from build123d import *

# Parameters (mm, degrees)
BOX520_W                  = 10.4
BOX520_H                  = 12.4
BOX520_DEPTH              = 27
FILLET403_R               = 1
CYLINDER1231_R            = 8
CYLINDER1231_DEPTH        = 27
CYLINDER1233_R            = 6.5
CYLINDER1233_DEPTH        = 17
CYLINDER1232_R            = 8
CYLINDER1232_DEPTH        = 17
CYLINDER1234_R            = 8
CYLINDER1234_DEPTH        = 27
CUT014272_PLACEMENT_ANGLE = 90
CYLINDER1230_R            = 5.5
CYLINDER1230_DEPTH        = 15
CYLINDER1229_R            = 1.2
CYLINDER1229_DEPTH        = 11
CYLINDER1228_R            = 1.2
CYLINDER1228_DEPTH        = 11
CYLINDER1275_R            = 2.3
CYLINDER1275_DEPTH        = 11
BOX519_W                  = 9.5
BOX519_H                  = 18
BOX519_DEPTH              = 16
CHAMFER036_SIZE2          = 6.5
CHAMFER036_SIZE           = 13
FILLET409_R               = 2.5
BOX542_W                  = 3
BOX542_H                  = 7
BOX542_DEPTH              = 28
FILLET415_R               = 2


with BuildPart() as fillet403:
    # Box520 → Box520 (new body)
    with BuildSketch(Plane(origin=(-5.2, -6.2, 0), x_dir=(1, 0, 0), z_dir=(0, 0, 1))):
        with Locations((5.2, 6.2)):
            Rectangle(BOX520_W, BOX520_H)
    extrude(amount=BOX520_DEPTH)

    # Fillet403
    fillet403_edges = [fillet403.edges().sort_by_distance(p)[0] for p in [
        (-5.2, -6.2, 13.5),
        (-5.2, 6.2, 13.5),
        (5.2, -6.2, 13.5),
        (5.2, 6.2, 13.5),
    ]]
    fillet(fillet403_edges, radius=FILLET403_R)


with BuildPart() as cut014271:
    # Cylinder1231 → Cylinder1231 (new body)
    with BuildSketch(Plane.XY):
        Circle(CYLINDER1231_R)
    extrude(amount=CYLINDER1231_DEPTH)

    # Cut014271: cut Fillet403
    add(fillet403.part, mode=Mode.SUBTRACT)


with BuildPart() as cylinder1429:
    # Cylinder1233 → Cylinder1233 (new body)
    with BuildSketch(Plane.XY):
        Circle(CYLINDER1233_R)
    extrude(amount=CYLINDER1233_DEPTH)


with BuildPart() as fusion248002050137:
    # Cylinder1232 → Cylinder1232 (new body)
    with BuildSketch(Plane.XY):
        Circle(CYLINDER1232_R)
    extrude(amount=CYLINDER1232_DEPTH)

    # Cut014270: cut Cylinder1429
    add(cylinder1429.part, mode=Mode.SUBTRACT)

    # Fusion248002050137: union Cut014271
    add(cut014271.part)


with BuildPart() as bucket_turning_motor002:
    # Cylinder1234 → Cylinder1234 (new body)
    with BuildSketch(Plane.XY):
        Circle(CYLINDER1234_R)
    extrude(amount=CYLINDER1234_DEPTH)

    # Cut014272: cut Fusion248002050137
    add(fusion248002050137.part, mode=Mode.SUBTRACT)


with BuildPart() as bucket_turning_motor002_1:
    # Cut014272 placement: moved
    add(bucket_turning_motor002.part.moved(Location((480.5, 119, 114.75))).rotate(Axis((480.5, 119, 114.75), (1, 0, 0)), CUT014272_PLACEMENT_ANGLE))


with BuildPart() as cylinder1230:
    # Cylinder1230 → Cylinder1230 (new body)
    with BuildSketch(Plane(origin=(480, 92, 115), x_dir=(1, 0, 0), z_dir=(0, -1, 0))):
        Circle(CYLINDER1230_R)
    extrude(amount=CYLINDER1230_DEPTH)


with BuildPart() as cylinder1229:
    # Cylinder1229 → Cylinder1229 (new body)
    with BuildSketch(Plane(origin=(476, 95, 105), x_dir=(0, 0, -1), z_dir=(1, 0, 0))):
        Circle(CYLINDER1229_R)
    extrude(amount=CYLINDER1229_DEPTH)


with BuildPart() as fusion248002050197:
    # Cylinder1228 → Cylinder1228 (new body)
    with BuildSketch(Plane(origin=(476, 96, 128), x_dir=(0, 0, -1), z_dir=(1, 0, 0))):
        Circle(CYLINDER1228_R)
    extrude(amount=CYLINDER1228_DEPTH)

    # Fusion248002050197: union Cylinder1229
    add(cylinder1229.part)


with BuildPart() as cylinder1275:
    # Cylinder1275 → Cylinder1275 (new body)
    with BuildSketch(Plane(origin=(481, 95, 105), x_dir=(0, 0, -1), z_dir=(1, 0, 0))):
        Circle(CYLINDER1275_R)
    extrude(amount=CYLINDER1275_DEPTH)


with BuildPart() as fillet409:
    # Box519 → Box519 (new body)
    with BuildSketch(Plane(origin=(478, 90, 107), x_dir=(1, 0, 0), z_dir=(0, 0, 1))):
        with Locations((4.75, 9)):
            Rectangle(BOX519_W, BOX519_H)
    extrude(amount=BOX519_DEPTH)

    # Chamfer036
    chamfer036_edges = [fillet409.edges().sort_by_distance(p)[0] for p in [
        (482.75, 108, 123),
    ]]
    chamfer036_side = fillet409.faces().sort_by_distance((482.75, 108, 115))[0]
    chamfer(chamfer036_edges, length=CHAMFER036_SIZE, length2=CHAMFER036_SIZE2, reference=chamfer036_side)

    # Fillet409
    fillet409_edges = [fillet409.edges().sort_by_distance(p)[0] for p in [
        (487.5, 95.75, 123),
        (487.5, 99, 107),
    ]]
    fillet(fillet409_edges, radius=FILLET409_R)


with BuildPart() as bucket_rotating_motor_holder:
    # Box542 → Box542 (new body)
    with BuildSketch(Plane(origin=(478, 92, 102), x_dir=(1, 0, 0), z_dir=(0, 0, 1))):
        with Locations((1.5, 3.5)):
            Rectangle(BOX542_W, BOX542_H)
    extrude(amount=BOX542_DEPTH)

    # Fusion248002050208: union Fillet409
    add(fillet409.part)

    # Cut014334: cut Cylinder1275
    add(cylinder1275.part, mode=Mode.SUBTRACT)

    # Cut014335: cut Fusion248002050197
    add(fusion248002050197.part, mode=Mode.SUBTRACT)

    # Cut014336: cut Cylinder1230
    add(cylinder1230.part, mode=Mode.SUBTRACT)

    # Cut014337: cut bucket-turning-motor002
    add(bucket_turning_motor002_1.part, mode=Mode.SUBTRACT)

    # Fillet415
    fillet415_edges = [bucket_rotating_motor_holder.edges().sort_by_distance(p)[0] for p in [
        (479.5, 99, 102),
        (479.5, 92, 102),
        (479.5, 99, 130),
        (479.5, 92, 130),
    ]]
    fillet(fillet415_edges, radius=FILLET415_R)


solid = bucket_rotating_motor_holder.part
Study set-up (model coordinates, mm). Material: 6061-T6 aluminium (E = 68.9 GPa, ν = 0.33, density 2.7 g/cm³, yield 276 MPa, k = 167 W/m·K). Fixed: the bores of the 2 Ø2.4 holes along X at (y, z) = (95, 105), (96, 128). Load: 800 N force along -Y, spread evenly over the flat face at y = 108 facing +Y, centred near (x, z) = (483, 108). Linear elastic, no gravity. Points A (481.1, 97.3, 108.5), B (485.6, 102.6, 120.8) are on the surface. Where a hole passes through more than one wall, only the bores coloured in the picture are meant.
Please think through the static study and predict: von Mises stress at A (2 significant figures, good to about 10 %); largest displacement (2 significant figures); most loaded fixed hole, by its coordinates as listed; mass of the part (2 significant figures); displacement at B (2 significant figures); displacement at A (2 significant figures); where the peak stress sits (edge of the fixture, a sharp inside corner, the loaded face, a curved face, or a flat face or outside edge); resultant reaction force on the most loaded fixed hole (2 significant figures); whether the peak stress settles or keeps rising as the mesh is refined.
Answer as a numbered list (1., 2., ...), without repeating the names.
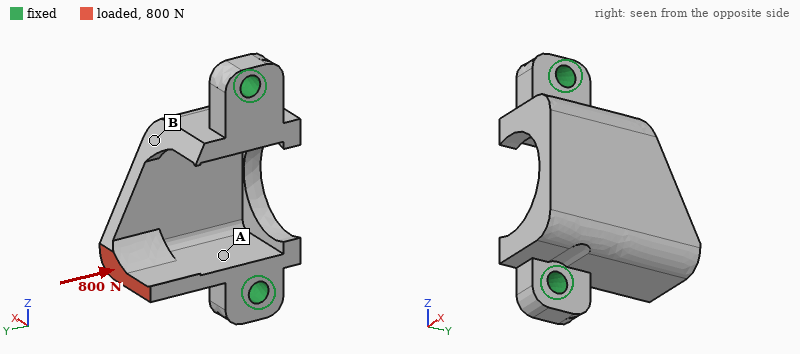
1. 65 MPa
2. 78 µm
3. (95, 105)
4. 3.0 g
5. 34 µm
6. 15 µm
7. edge of the fixture
8. 730 N
9. keeps rising
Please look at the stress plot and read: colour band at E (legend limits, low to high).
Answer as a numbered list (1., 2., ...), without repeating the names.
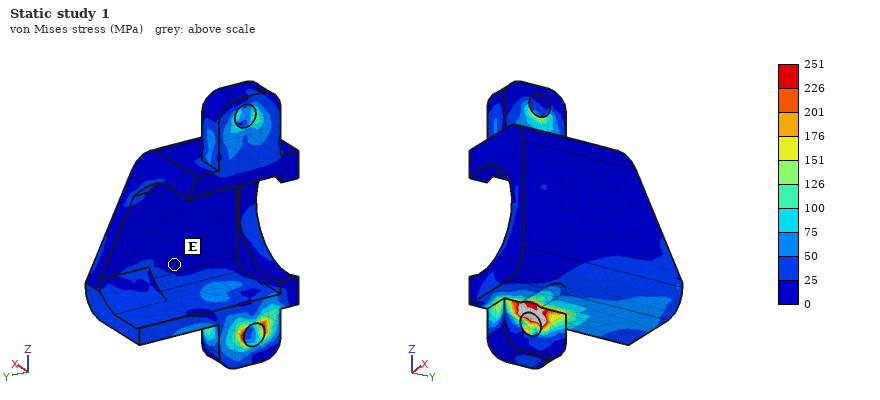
1. 0 to 25 MPa
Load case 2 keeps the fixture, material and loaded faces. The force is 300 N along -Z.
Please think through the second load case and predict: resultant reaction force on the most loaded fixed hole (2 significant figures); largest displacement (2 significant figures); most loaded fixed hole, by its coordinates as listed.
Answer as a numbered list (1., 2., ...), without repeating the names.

1. 260 N
2. 0.14 mm
3. (95, 105)
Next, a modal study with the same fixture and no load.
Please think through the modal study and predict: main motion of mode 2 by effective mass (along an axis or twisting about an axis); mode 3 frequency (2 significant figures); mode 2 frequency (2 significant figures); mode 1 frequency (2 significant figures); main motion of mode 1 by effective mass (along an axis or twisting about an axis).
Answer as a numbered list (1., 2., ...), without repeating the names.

1. along Z
2. 24 kHz
3. 15 kHz
4. 11 kHz
5. along Y
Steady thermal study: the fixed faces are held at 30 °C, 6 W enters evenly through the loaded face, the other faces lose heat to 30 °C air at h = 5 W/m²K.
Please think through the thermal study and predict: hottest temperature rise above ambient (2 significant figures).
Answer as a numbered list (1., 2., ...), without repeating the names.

1. 23 K
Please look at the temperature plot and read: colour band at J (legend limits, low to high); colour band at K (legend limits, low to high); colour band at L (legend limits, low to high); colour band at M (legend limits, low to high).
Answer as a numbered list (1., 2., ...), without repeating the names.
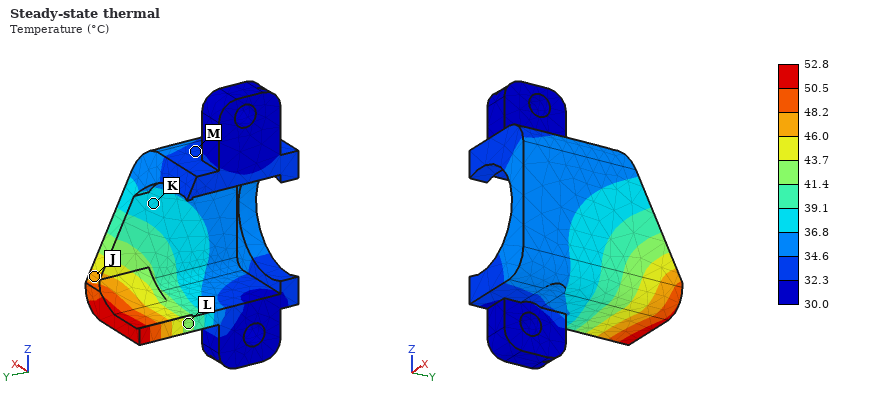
1. 46.0 to 48.2 °C
2. 36.8 to 39.1 °C
3. 41.4 to 43.7 °C
4. 32.3 to 34.6 °C
